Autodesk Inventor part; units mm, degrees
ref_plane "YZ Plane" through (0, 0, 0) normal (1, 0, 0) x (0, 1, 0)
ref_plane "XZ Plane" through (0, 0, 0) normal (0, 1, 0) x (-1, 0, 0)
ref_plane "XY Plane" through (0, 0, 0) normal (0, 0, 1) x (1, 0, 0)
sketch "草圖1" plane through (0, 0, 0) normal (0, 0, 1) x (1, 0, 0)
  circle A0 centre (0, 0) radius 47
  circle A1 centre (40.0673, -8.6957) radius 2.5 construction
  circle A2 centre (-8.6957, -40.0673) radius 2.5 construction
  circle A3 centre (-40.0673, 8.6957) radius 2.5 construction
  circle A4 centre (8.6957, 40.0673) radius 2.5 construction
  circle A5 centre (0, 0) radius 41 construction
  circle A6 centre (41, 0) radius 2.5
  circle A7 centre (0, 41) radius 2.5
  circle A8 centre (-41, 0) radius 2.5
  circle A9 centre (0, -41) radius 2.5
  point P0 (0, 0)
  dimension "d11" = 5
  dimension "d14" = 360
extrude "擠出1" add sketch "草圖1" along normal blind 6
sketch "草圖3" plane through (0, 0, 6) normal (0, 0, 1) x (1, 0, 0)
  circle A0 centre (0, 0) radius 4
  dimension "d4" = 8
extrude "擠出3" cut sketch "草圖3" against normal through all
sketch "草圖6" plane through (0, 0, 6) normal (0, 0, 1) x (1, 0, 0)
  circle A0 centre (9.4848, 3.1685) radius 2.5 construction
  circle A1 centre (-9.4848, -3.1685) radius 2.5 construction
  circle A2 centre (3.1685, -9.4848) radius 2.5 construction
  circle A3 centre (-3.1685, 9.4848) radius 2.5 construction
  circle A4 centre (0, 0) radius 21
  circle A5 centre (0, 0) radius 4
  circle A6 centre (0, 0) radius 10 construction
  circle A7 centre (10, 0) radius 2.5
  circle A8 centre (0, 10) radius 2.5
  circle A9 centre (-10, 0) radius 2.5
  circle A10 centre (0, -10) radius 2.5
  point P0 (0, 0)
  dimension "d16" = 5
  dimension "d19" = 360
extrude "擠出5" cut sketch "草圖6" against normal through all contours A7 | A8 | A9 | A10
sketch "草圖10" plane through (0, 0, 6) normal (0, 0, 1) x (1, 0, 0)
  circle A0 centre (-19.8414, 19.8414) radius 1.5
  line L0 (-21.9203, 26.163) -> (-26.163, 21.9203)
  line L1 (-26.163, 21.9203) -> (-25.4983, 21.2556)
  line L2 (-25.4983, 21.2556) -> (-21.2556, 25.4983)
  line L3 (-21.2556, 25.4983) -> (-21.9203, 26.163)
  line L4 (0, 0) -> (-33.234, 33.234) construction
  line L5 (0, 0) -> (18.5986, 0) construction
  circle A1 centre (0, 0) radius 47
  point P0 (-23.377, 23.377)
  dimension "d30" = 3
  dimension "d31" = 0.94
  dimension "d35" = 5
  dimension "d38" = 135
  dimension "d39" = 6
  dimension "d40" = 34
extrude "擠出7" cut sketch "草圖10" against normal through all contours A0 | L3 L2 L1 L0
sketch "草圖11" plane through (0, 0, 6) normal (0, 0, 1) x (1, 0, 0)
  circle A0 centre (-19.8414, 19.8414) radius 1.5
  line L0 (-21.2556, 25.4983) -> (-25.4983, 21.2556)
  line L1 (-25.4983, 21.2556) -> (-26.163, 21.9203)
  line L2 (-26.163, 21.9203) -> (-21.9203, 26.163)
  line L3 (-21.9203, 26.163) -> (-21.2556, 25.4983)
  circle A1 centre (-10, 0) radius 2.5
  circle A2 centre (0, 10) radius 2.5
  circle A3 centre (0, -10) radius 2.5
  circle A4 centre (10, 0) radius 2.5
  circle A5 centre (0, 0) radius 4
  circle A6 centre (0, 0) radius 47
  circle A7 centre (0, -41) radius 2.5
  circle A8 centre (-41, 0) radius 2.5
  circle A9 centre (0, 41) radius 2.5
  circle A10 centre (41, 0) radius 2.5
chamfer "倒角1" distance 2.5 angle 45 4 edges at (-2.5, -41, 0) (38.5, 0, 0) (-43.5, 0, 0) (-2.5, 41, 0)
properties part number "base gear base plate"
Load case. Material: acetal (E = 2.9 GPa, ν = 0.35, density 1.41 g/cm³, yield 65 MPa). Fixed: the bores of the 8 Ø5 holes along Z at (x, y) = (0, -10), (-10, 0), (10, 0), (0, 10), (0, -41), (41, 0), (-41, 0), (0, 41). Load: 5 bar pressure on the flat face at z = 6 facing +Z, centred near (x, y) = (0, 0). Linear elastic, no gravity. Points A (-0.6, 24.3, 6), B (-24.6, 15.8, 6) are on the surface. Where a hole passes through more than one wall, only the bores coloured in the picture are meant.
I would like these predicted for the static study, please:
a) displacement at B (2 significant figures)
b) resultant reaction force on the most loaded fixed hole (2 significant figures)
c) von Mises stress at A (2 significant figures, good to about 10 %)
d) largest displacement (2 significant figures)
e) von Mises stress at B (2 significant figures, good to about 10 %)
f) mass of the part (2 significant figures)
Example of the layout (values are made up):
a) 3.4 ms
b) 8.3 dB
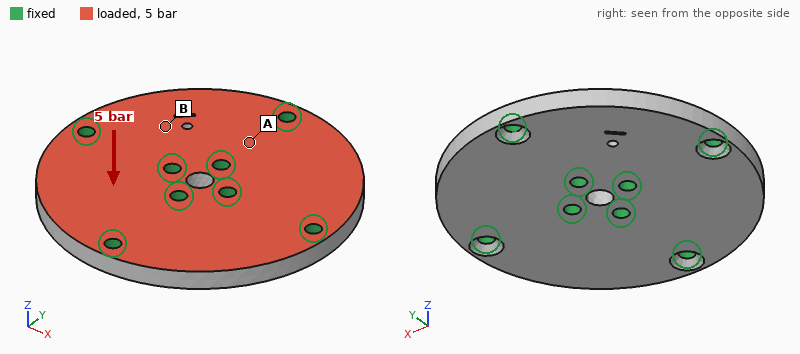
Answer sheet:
a) 0.21 mm
b) 540 N
c) 11 MPa
d) 0.54 mm
e) 5.6 MPa
f) 56 g
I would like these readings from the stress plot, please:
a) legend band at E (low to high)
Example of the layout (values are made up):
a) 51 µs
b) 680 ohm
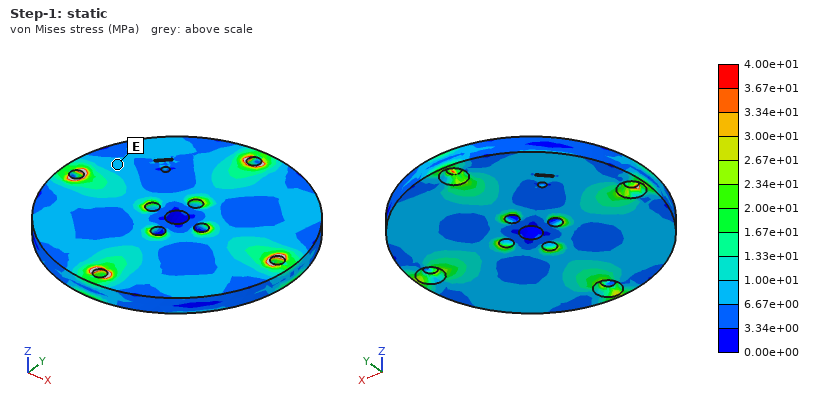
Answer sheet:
a) 6.67e+00 to 1.00e+01 MPa
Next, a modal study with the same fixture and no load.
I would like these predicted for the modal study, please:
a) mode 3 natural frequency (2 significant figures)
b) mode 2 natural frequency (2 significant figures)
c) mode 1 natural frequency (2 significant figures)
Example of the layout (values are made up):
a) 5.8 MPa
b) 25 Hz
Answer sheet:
a) 2100 Hz
b) 2100 Hz
c) 1900 Hz
